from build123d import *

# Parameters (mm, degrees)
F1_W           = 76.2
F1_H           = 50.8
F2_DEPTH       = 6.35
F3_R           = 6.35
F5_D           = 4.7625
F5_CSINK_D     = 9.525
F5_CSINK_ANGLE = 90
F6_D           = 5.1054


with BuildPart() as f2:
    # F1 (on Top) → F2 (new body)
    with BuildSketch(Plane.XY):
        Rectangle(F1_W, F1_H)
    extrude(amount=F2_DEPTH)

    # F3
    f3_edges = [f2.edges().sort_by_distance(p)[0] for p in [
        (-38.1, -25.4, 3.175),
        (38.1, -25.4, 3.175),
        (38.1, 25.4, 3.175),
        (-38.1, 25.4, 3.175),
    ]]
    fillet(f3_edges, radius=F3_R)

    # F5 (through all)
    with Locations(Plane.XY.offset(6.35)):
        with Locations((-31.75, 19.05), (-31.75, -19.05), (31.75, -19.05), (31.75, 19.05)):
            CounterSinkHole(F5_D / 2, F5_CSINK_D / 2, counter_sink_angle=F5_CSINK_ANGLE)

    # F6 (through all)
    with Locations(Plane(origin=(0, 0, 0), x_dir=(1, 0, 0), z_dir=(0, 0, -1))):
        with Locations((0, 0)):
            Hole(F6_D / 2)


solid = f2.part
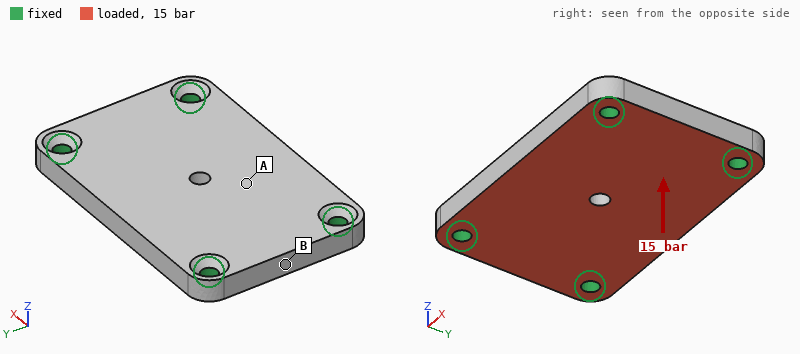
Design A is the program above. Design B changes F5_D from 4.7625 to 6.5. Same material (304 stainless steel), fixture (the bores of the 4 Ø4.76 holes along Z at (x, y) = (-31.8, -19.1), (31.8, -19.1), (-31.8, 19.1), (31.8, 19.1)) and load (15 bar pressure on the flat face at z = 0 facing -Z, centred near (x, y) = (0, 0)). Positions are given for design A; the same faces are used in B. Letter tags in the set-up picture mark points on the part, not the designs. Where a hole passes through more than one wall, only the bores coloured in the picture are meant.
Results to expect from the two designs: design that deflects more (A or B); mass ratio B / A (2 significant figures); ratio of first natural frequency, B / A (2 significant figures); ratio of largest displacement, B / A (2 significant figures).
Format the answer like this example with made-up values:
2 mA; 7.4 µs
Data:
A; 0.99; 1.2; 0.77
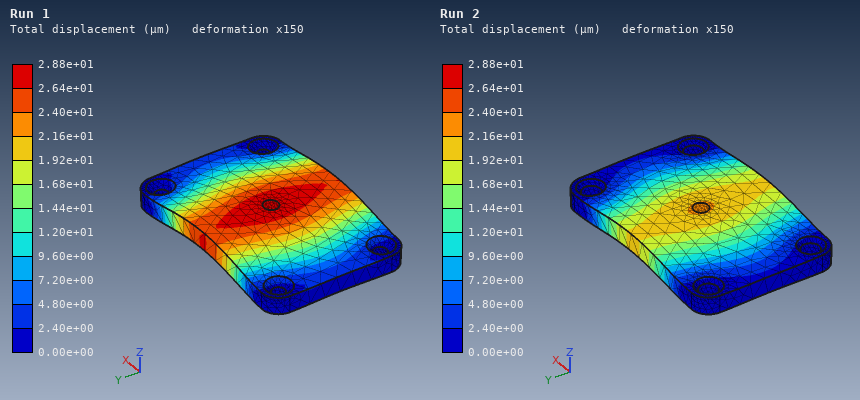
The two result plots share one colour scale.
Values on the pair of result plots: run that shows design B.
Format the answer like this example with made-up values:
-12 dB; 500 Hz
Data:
Run 2
